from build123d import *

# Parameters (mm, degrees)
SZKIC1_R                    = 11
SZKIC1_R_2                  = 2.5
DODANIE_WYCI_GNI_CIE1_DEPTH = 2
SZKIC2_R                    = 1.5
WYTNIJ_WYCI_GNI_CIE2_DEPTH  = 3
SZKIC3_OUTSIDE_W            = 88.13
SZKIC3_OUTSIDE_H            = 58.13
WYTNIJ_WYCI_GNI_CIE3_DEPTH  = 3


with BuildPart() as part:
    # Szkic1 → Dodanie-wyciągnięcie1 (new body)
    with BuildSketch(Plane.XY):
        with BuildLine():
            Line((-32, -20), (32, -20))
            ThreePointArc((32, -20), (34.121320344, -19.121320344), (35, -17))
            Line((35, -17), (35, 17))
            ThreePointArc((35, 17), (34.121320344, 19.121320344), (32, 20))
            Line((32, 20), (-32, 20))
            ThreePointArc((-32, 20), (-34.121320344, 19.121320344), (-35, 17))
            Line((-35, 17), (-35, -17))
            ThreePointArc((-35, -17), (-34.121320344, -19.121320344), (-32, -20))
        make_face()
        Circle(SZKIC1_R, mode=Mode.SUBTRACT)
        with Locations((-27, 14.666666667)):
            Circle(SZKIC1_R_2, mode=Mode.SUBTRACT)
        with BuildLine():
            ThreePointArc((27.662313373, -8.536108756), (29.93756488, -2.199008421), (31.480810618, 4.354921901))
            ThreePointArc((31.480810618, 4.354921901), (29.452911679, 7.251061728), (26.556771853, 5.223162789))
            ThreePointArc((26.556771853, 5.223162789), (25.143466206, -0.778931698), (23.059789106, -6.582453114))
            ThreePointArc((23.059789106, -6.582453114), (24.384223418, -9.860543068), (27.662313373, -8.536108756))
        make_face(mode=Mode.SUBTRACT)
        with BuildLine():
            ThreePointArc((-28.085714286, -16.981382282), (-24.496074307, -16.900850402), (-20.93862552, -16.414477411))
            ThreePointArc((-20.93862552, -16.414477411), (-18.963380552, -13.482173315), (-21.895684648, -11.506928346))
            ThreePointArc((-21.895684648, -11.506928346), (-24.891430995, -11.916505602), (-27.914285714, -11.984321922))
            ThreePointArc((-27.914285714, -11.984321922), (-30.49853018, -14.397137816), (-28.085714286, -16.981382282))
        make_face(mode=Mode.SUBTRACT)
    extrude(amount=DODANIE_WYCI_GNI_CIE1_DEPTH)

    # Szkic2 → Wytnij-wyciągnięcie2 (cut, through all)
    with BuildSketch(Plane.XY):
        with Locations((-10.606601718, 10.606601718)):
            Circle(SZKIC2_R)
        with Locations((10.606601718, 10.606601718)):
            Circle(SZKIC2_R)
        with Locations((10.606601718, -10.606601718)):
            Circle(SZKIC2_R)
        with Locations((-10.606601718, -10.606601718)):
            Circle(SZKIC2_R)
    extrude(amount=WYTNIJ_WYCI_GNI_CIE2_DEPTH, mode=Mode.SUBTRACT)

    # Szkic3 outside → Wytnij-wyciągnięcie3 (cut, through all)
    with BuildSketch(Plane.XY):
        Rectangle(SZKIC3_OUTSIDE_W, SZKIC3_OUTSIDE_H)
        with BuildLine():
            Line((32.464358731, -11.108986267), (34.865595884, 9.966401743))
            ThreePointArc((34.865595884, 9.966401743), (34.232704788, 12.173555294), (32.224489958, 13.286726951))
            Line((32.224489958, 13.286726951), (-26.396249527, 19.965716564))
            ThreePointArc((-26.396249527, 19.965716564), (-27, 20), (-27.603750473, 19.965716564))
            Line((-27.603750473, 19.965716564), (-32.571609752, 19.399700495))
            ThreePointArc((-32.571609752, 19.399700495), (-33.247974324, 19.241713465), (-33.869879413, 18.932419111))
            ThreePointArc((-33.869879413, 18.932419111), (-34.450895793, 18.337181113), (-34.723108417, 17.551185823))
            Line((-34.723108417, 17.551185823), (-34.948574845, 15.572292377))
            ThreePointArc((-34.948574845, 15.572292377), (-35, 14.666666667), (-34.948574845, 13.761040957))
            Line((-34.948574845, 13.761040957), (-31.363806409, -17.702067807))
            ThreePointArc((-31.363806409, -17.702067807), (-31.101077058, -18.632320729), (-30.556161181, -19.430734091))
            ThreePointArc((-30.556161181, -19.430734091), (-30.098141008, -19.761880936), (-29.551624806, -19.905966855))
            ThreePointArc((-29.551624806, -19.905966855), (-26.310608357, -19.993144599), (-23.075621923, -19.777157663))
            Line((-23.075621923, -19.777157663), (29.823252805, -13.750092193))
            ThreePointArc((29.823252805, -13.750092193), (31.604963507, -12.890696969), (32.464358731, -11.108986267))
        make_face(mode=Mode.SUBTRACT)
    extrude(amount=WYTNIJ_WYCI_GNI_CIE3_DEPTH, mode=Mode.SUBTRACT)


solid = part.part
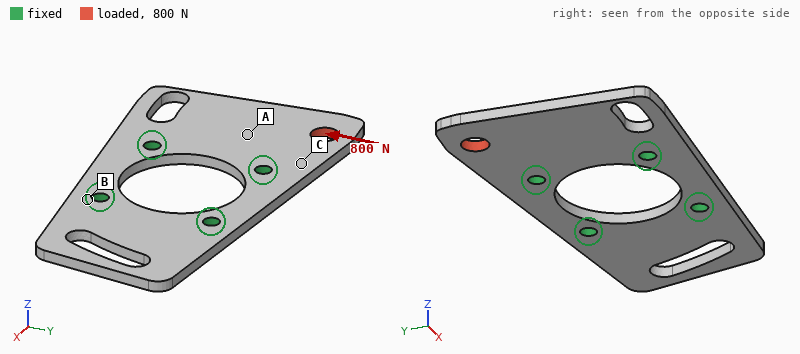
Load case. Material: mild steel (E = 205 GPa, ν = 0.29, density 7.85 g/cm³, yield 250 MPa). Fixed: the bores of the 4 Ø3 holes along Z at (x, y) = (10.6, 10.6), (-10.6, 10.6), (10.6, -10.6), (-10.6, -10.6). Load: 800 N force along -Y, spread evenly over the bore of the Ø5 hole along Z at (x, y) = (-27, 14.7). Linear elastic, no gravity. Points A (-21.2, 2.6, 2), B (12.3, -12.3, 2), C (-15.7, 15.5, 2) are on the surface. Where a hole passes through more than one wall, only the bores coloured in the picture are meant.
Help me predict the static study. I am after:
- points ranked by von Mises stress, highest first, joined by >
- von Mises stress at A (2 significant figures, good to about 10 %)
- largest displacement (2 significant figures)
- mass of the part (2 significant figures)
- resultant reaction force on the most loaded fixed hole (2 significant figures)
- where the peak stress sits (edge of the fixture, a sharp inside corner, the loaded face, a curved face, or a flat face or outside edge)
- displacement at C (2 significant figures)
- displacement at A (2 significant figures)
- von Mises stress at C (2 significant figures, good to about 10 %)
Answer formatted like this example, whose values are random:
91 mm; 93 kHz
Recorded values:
A > C > B; 29 MPa; 7.6 µm; 27 g; 630 N; edge of the fixture; 2.2 µm; 2.7 µm; 16 MPa
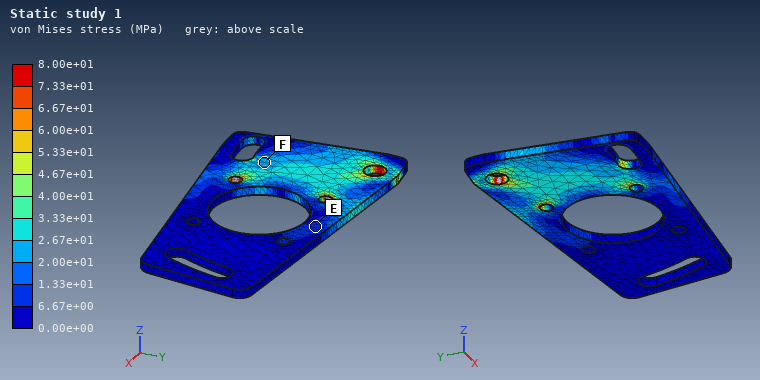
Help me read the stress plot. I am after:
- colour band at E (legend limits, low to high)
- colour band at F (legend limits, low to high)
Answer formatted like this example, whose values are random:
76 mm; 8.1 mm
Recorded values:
6.67e+00 to 1.33e+01 MPa; 2.00e+01 to 2.67e+01 MPa
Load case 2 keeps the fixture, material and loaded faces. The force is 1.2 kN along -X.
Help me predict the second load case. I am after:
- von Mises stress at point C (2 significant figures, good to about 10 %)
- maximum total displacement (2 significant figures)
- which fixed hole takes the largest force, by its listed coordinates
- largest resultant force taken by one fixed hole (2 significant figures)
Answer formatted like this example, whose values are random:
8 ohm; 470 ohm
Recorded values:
53 MPa; 8.8 µm; (-10.6, 10.6); 1.2 kN
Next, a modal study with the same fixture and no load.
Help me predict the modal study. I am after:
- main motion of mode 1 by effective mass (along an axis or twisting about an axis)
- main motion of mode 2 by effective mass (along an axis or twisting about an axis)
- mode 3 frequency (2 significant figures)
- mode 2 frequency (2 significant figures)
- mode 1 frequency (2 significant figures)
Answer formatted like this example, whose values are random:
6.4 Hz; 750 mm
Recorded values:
along Z; along Z; 5600 Hz; 3400 Hz; 3000 Hz
